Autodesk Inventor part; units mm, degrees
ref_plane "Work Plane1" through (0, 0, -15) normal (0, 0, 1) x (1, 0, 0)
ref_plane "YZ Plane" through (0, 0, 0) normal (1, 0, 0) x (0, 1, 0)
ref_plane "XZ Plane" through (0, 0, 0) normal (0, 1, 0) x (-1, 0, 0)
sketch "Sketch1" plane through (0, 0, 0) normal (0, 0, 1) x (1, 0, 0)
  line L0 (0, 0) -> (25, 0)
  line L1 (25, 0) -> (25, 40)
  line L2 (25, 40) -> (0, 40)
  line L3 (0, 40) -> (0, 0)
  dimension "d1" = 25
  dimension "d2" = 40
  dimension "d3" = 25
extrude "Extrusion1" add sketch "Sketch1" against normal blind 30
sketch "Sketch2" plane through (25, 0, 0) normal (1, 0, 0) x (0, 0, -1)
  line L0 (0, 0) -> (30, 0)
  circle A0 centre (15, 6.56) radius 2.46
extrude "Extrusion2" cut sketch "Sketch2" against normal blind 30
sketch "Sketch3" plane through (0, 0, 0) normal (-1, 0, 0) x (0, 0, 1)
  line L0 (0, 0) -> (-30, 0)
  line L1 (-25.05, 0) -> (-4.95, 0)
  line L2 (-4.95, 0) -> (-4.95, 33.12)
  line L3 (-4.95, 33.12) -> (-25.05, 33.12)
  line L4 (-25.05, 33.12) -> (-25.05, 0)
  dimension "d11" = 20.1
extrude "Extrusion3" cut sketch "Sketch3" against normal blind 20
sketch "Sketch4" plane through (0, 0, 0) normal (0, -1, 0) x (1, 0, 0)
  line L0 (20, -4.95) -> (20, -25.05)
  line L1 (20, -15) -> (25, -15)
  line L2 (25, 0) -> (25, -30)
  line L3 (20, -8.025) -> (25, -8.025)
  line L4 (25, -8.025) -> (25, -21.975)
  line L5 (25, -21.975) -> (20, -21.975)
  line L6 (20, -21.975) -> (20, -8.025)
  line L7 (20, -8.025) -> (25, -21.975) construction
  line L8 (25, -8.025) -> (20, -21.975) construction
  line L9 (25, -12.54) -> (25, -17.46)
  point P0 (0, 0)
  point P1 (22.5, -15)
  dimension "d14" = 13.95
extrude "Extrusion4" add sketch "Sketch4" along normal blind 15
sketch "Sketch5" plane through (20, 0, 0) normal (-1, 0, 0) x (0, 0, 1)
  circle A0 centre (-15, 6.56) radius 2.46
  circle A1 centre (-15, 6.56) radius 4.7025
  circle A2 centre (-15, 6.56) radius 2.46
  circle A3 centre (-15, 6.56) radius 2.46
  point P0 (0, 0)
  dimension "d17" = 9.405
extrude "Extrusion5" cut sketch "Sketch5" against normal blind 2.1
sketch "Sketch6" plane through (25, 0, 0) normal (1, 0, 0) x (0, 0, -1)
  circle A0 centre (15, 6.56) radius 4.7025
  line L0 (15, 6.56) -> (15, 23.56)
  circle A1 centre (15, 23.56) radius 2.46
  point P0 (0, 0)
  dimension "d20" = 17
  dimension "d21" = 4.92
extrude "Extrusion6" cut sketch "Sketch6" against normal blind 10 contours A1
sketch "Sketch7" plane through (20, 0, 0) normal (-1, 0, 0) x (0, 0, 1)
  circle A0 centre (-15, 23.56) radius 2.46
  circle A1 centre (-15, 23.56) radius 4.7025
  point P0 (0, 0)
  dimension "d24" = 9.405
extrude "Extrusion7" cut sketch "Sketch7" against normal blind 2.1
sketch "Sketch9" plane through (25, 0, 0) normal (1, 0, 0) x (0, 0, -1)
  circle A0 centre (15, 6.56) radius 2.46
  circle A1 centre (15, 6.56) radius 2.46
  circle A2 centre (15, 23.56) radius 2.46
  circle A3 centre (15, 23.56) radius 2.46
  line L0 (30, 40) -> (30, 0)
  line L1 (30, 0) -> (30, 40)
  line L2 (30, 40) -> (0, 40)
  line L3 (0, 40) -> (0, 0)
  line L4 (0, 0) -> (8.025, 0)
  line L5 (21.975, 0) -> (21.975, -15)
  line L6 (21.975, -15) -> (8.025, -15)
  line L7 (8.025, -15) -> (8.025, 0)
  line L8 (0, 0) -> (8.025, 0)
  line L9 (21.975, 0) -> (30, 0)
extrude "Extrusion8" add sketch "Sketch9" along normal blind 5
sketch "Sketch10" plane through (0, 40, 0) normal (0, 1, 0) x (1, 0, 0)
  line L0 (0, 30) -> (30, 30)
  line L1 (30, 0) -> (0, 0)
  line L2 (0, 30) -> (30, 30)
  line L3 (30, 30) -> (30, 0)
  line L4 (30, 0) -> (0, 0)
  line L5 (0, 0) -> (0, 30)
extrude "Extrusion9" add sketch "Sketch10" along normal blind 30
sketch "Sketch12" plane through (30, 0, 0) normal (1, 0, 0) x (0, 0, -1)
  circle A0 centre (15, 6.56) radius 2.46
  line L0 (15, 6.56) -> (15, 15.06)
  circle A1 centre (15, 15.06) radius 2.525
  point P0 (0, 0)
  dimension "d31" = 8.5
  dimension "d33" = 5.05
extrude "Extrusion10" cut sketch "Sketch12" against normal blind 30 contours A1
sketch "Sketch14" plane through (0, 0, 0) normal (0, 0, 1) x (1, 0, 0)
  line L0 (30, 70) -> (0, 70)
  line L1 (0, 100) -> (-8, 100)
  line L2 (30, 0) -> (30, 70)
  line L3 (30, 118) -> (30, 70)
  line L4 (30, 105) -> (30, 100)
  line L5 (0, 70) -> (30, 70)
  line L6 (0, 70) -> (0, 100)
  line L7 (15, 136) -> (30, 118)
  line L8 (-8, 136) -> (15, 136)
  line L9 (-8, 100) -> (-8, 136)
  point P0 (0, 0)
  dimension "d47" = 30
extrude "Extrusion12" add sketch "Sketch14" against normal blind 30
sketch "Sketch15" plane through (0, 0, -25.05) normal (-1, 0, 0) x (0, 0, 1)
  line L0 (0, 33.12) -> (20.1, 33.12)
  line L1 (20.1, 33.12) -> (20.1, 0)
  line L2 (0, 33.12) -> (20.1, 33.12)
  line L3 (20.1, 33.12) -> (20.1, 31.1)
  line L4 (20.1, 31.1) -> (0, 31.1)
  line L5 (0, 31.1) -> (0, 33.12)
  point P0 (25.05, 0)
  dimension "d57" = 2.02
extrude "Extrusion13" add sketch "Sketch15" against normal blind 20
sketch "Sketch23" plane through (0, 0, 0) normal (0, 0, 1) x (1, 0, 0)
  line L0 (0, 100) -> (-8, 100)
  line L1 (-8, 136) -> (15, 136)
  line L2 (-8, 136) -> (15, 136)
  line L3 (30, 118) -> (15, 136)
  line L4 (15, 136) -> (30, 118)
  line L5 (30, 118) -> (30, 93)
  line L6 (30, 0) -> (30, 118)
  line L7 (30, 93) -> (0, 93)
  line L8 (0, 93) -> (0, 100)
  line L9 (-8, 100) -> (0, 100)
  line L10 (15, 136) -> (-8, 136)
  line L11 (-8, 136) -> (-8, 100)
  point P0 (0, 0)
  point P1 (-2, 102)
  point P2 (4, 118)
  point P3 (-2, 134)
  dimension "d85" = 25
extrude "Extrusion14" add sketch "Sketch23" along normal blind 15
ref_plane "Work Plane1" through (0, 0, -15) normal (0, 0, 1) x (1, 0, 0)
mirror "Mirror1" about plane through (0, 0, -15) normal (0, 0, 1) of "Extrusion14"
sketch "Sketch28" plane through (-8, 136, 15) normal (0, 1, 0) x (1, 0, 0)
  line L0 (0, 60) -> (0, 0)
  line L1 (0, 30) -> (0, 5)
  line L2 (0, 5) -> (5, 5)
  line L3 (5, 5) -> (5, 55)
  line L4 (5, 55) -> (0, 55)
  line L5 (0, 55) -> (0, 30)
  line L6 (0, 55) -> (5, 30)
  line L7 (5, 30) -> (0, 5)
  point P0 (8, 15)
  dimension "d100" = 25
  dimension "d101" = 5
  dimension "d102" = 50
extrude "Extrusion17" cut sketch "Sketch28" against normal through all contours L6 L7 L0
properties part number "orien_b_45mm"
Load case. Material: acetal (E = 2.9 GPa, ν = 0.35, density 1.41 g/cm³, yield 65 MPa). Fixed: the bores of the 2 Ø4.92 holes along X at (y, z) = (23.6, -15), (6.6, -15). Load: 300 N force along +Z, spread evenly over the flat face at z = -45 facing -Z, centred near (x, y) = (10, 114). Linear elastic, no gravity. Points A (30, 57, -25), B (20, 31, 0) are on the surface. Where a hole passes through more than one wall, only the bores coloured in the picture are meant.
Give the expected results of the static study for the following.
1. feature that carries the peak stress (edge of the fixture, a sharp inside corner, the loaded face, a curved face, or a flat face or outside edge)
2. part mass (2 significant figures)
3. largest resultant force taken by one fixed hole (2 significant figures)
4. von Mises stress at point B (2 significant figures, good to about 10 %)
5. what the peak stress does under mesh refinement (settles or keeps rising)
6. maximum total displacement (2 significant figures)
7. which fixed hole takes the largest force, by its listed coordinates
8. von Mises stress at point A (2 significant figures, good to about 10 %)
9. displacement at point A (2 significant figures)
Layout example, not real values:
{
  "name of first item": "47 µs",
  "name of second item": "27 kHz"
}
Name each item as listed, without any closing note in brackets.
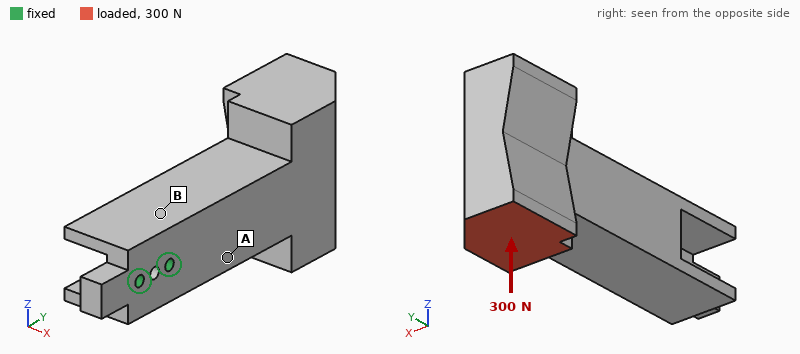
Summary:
{
  "feature that carries the peak stress": "edge of the fixture",
  "part mass": "220 g",
  "largest resultant force taken by one fixed hole": "1.5 kN",
  "von Mises stress at point B": "9.7 MPa",
  "what the peak stress does under mesh refinement": "keeps rising",
  "maximum total displacement": "1.7 mm",
  "which fixed hole takes the largest force, by its listed coordinates": "(23.6, -15)",
  "von Mises stress at point A": "2.8 MPa",
  "displacement at point A": "0.37 mm"
}
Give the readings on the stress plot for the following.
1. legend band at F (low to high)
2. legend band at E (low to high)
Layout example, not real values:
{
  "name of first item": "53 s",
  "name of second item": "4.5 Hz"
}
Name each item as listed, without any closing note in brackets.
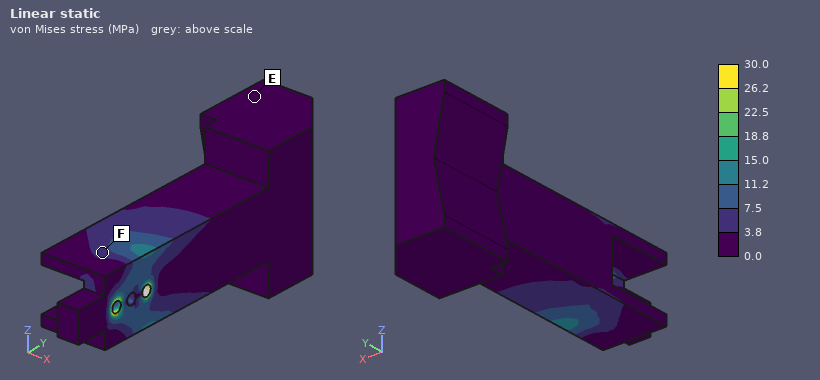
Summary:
{
  "legend band at F": "3.8 to 7.5 MPa",
  "legend band at E": "0.0 to 3.8 MPa"
}
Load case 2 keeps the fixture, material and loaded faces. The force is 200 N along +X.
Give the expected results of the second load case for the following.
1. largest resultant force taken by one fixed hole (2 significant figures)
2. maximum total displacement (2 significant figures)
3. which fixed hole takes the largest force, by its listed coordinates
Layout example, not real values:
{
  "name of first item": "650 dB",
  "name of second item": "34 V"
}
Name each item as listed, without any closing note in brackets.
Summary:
{
  "largest resultant force taken by one fixed hole": "920 N",
  "maximum total displacement": "1.7 mm",
  "which fixed hole takes the largest force, by its listed coordinates": "(23.6, -15)"
}
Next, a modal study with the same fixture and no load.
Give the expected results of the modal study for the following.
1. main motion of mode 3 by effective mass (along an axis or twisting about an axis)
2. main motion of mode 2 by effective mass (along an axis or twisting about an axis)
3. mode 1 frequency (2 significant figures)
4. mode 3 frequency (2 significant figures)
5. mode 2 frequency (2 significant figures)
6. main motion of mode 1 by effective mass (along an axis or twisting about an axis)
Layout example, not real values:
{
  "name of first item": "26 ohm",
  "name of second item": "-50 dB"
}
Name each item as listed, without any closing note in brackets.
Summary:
{
  "main motion of mode 3 by effective mass": "twisting about Y",
  "main motion of mode 2 by effective mass": "along Z",
  "mode 1 frequency": "180 Hz",
  "mode 3 frequency": "510 Hz",
  "mode 2 frequency": "210 Hz",
  "main motion of mode 1 by effective mass": "along X"
}
